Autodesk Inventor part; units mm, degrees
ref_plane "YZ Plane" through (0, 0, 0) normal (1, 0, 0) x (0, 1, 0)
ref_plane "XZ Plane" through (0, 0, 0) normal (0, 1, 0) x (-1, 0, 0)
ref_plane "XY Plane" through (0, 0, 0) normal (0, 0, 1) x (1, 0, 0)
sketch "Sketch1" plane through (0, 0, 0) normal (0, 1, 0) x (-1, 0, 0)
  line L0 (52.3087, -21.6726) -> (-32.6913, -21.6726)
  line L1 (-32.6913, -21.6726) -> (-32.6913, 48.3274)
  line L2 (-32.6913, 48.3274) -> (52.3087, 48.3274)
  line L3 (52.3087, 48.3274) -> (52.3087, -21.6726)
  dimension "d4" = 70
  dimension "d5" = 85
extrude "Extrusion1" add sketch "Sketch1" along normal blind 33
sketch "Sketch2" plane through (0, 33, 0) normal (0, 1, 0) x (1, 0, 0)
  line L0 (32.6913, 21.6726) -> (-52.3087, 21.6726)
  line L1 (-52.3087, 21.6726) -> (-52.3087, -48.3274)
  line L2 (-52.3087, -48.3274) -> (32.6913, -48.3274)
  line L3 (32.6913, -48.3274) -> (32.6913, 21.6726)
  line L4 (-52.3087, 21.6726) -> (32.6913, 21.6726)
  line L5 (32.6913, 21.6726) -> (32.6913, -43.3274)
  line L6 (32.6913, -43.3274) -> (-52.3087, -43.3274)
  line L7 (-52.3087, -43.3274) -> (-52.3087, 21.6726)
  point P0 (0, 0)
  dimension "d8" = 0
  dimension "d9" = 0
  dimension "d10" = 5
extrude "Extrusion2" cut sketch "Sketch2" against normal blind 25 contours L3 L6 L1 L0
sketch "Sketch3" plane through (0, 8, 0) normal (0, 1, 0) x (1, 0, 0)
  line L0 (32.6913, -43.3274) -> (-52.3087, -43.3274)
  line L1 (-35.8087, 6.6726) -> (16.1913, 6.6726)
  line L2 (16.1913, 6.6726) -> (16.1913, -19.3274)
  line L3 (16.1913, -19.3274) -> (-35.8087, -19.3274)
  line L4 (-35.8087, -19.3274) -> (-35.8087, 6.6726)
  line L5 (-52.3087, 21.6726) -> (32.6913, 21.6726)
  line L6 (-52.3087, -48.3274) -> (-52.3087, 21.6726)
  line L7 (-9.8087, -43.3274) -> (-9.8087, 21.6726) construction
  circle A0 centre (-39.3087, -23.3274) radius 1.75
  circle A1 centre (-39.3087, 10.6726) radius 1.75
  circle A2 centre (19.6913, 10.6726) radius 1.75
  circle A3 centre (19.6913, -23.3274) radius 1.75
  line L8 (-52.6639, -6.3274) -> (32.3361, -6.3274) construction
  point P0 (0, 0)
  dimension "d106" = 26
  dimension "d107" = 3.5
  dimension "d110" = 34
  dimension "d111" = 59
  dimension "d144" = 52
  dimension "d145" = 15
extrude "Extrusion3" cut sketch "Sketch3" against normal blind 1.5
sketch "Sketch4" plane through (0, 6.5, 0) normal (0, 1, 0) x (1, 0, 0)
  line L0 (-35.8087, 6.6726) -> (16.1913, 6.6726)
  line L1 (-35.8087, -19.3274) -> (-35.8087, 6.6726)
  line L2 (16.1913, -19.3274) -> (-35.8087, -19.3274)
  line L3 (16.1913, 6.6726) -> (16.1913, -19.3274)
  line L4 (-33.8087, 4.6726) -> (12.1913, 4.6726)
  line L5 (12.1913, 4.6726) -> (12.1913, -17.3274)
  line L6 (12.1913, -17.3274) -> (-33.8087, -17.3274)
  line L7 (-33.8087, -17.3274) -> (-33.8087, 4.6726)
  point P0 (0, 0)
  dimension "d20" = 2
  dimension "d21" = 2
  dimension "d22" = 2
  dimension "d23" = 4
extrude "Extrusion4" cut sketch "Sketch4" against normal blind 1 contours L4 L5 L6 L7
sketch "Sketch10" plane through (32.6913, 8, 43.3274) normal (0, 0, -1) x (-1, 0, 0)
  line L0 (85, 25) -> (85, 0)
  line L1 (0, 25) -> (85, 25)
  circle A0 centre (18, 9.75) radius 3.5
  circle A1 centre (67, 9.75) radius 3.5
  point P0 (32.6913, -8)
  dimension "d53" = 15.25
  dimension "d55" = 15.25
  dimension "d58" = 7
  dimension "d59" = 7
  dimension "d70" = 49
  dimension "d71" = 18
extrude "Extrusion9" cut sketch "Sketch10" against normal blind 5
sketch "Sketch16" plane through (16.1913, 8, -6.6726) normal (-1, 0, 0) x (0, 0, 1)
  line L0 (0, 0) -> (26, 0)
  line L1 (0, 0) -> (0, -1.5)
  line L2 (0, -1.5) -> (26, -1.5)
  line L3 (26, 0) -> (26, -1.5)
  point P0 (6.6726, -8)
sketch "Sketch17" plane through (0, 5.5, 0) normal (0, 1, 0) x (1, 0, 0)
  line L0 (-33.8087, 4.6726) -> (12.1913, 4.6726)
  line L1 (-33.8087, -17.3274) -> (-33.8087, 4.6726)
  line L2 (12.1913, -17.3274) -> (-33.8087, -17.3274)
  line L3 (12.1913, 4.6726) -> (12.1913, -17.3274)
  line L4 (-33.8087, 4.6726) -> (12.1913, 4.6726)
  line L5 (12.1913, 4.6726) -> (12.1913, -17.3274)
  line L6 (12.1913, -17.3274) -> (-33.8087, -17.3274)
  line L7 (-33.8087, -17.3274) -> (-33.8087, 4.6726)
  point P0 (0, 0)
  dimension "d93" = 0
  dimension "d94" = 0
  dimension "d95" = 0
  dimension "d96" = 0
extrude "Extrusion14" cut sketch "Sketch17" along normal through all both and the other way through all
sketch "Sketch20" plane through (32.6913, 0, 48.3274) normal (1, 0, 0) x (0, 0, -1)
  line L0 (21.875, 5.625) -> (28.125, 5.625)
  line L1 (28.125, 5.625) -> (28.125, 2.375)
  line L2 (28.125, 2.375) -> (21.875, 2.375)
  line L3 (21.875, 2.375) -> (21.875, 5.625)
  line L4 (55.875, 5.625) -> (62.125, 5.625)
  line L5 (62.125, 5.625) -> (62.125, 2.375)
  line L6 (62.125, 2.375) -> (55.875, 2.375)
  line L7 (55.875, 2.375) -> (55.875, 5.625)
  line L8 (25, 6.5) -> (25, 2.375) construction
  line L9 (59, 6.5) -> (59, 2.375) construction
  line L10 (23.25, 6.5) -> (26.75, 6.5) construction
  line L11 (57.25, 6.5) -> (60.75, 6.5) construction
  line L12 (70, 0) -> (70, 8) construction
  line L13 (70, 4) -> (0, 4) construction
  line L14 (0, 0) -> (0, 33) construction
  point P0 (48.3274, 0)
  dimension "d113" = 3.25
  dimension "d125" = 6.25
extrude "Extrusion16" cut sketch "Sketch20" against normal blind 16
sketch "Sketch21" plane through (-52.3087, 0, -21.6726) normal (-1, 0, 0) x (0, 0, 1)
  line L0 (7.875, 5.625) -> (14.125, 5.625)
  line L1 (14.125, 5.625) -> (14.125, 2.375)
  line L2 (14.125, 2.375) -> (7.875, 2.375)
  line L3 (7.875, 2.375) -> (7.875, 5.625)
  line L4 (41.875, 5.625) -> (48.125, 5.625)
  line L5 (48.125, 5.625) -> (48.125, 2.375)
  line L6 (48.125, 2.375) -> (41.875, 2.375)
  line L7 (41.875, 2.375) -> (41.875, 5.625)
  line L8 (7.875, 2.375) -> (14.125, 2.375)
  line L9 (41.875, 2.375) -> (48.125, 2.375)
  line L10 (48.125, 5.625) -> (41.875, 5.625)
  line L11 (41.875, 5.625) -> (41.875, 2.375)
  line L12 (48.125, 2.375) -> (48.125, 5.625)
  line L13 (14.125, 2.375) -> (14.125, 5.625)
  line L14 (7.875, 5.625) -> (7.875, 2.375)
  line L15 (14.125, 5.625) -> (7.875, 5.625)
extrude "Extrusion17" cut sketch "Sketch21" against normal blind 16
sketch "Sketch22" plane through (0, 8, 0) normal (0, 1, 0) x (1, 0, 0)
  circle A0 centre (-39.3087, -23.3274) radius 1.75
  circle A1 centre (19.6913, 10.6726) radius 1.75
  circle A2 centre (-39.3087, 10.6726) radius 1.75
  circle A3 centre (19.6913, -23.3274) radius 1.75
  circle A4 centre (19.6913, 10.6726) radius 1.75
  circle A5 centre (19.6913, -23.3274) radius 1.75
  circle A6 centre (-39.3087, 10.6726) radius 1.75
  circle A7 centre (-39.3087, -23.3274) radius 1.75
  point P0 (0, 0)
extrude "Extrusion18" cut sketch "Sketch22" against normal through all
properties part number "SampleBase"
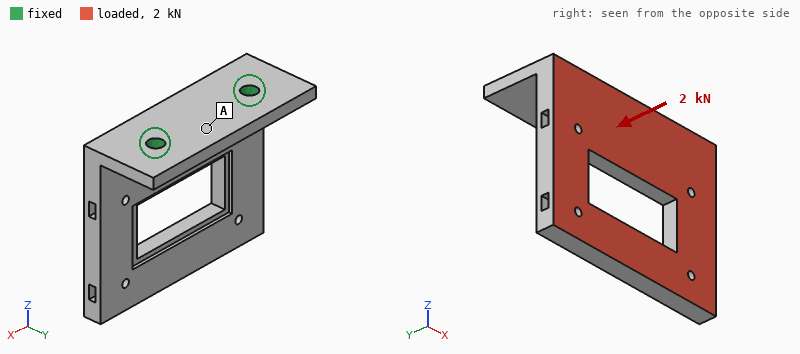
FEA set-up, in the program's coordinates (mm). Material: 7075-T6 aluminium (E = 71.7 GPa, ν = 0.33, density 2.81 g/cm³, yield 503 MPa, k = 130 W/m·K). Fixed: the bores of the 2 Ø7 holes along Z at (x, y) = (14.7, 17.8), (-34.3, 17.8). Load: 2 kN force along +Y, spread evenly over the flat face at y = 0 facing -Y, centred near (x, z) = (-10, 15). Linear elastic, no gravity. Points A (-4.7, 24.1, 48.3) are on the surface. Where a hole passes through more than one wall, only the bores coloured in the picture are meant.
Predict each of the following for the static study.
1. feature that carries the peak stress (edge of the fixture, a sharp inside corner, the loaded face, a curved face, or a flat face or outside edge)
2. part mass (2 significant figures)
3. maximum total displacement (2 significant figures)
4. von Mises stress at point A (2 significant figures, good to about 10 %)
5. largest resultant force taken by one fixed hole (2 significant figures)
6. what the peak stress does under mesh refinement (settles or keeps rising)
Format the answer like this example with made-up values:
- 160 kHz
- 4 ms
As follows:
- edge of the fixture
- 130 g
- 1.2 mm
- 34 MPa
- 1.0 kN
- keeps rising
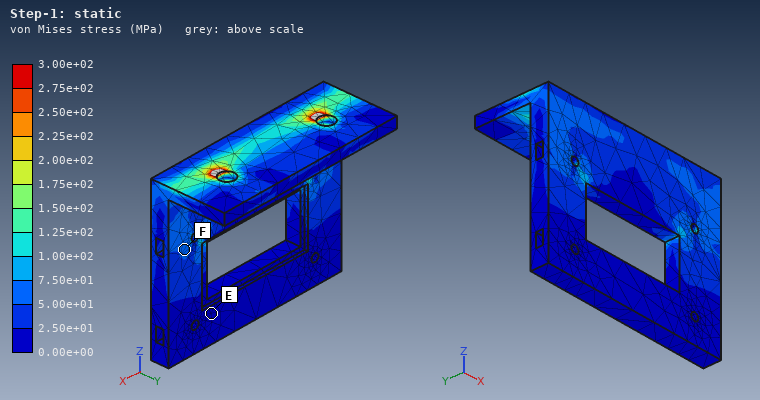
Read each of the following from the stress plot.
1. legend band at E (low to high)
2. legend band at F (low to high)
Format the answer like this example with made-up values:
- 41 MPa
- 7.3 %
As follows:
- 0.00e+00 to 2.50e+01 MPa
- 5.00e+01 to 7.50e+01 MPa
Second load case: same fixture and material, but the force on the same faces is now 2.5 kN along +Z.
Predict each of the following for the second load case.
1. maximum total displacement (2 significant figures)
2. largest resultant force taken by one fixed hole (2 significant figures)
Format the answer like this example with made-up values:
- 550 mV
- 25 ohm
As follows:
- 0.46 mm
- 1.3 kN
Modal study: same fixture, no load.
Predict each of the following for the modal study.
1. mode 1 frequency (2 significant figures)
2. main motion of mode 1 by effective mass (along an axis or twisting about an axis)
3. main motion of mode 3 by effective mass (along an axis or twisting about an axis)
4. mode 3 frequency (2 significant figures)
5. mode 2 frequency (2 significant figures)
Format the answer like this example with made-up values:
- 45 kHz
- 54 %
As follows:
- 780 Hz
- along Y
- along X
- 3100 Hz
- 1900 Hz
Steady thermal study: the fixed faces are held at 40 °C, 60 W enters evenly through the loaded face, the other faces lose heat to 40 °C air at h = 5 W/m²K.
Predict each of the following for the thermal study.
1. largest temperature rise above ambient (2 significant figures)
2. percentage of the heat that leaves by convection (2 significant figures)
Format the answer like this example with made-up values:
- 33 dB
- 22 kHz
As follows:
- 56 K
- 3.2 %
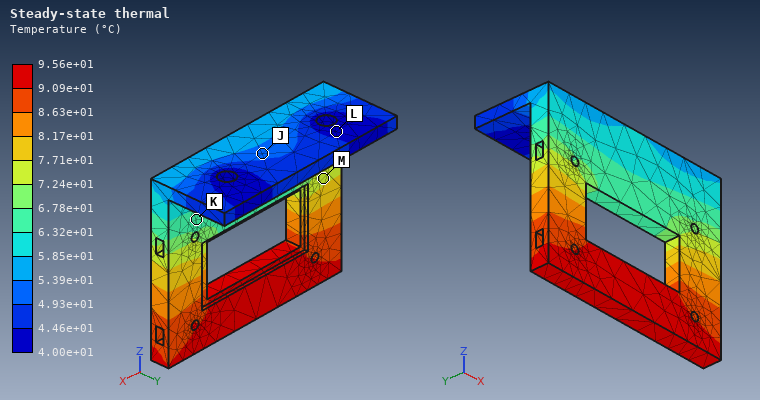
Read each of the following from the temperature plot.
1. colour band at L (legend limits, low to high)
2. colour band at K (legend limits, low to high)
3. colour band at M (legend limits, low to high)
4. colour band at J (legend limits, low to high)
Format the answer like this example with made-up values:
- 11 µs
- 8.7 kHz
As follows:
- 4.00e+01 to 4.46e+01 °C
- 6.32e+01 to 6.78e+01 °C
- 7.24e+01 to 7.71e+01 °C
- 4.93e+01 to 5.39e+01 °C
